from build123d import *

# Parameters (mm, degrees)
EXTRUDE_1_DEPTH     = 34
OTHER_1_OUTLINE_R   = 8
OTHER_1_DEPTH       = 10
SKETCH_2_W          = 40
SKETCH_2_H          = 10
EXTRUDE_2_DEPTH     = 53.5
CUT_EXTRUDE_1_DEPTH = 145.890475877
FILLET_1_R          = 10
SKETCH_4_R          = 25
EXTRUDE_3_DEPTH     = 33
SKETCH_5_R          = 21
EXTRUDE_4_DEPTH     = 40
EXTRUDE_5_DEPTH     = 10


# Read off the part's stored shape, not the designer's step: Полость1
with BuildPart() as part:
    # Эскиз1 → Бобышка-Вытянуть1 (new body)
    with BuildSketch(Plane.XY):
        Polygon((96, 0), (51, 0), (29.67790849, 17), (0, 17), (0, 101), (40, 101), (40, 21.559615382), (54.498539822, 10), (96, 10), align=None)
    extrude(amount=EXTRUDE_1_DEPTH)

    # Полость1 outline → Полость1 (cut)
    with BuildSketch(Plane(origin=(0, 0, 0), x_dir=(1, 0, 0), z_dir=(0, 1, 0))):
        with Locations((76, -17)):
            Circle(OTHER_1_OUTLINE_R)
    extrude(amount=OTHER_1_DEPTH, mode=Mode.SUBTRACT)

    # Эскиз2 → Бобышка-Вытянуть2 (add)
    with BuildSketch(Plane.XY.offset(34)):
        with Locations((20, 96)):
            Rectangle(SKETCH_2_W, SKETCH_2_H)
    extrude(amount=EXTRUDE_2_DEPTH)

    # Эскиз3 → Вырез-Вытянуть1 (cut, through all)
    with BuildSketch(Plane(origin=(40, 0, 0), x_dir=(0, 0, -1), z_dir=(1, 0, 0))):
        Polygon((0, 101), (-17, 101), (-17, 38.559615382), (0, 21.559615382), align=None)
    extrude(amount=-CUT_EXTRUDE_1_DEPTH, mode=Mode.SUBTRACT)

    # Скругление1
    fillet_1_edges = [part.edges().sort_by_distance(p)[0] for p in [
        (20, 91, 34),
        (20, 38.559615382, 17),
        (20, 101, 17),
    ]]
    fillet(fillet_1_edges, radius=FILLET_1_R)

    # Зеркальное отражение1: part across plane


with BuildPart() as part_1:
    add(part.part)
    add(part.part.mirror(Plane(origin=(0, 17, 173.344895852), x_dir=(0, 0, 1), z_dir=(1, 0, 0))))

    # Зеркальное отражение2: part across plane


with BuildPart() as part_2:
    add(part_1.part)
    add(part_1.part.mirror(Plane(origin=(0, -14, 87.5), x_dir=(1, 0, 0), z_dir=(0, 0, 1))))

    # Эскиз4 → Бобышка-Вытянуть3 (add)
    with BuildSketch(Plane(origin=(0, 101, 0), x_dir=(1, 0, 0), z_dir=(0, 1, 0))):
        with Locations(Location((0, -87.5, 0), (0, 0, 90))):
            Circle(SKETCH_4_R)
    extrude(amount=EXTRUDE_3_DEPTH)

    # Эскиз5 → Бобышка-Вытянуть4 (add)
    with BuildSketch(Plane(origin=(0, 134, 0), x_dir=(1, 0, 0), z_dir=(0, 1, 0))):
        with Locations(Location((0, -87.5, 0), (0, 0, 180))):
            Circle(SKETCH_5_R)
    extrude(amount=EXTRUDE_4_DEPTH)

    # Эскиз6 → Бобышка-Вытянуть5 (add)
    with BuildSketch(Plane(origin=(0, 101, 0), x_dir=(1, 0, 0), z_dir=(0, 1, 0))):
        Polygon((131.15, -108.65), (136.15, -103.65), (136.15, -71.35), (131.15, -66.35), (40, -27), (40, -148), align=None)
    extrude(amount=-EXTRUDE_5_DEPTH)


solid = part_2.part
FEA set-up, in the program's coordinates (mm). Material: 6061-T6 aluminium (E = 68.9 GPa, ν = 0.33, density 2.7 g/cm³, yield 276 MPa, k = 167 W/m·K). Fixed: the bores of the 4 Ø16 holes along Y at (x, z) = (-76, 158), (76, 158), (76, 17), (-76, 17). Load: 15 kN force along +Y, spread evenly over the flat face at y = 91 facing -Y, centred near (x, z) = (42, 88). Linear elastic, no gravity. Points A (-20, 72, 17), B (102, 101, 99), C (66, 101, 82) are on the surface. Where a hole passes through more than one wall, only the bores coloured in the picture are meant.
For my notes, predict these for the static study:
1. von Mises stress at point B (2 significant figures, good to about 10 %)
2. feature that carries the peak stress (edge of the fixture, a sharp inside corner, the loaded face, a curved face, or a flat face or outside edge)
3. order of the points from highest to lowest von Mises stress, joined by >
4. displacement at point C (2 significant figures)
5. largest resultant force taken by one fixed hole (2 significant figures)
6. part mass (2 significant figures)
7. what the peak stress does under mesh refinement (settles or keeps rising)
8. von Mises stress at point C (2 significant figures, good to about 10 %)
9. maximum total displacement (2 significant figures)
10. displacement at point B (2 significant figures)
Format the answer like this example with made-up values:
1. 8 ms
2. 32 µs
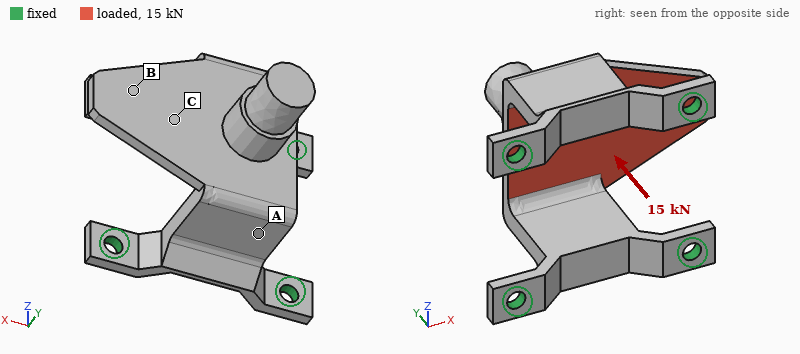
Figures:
1. 56 MPa
2. a sharp inside corner
3. C > B > A
4. 0.86 mm
5. 8.5 kN
6. 1.7 kg
7. keeps rising
8. 110 MPa
9. 2.6 mm
10. 1.7 mm
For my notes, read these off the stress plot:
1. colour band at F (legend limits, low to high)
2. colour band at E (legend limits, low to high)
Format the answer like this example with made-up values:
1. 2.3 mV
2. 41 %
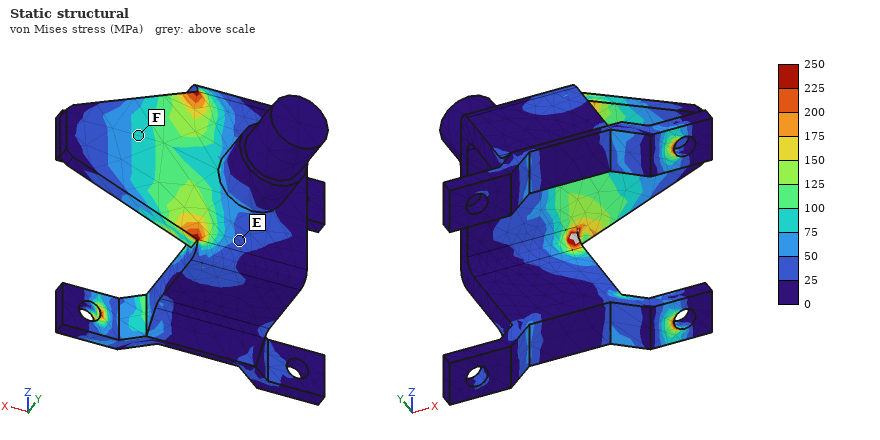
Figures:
1. 75 to 100 MPa
2. 25 to 50 MPa
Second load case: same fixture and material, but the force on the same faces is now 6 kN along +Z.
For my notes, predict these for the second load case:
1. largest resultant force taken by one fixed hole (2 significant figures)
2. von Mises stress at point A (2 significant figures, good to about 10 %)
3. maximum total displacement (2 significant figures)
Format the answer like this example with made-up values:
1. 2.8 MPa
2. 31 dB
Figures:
1. 3.4 kN
2. 16 MPa
3. 0.49 mm
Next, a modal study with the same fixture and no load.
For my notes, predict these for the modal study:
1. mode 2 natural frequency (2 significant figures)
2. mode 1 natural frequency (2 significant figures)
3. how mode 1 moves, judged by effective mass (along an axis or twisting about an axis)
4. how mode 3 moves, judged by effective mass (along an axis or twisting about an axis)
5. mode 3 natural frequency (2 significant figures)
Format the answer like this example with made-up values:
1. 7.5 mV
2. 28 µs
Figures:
1. 720 Hz
2. 640 Hz
3. along Z
4. along X
5. 1100 Hz
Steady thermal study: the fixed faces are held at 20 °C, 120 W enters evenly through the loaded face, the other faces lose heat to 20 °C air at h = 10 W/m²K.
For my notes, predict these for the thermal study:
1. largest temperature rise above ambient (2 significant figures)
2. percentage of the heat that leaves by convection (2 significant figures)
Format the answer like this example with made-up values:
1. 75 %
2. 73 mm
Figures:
1. 62 K
2. 21 %
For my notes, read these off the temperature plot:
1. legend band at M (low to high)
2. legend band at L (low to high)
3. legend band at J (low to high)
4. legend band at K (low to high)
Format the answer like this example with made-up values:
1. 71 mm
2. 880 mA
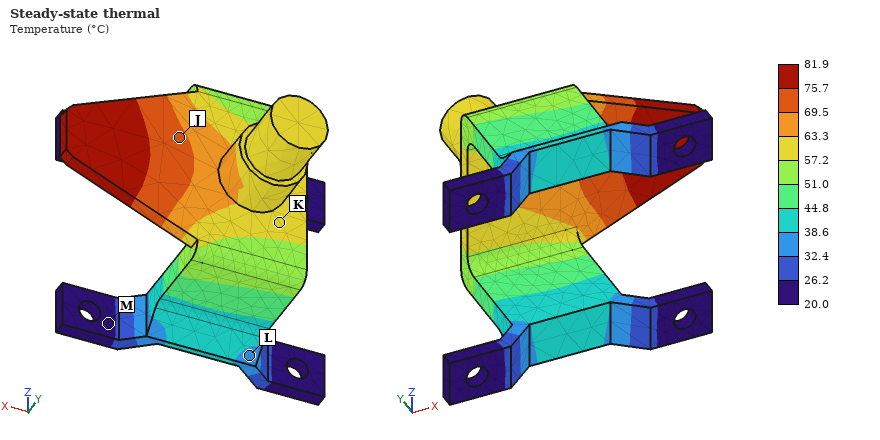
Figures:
1. 20.0 to 26.2 °C
2. 32.4 to 38.6 °C
3. 69.5 to 75.7 °C
4. 57.2 to 63.3 °C
